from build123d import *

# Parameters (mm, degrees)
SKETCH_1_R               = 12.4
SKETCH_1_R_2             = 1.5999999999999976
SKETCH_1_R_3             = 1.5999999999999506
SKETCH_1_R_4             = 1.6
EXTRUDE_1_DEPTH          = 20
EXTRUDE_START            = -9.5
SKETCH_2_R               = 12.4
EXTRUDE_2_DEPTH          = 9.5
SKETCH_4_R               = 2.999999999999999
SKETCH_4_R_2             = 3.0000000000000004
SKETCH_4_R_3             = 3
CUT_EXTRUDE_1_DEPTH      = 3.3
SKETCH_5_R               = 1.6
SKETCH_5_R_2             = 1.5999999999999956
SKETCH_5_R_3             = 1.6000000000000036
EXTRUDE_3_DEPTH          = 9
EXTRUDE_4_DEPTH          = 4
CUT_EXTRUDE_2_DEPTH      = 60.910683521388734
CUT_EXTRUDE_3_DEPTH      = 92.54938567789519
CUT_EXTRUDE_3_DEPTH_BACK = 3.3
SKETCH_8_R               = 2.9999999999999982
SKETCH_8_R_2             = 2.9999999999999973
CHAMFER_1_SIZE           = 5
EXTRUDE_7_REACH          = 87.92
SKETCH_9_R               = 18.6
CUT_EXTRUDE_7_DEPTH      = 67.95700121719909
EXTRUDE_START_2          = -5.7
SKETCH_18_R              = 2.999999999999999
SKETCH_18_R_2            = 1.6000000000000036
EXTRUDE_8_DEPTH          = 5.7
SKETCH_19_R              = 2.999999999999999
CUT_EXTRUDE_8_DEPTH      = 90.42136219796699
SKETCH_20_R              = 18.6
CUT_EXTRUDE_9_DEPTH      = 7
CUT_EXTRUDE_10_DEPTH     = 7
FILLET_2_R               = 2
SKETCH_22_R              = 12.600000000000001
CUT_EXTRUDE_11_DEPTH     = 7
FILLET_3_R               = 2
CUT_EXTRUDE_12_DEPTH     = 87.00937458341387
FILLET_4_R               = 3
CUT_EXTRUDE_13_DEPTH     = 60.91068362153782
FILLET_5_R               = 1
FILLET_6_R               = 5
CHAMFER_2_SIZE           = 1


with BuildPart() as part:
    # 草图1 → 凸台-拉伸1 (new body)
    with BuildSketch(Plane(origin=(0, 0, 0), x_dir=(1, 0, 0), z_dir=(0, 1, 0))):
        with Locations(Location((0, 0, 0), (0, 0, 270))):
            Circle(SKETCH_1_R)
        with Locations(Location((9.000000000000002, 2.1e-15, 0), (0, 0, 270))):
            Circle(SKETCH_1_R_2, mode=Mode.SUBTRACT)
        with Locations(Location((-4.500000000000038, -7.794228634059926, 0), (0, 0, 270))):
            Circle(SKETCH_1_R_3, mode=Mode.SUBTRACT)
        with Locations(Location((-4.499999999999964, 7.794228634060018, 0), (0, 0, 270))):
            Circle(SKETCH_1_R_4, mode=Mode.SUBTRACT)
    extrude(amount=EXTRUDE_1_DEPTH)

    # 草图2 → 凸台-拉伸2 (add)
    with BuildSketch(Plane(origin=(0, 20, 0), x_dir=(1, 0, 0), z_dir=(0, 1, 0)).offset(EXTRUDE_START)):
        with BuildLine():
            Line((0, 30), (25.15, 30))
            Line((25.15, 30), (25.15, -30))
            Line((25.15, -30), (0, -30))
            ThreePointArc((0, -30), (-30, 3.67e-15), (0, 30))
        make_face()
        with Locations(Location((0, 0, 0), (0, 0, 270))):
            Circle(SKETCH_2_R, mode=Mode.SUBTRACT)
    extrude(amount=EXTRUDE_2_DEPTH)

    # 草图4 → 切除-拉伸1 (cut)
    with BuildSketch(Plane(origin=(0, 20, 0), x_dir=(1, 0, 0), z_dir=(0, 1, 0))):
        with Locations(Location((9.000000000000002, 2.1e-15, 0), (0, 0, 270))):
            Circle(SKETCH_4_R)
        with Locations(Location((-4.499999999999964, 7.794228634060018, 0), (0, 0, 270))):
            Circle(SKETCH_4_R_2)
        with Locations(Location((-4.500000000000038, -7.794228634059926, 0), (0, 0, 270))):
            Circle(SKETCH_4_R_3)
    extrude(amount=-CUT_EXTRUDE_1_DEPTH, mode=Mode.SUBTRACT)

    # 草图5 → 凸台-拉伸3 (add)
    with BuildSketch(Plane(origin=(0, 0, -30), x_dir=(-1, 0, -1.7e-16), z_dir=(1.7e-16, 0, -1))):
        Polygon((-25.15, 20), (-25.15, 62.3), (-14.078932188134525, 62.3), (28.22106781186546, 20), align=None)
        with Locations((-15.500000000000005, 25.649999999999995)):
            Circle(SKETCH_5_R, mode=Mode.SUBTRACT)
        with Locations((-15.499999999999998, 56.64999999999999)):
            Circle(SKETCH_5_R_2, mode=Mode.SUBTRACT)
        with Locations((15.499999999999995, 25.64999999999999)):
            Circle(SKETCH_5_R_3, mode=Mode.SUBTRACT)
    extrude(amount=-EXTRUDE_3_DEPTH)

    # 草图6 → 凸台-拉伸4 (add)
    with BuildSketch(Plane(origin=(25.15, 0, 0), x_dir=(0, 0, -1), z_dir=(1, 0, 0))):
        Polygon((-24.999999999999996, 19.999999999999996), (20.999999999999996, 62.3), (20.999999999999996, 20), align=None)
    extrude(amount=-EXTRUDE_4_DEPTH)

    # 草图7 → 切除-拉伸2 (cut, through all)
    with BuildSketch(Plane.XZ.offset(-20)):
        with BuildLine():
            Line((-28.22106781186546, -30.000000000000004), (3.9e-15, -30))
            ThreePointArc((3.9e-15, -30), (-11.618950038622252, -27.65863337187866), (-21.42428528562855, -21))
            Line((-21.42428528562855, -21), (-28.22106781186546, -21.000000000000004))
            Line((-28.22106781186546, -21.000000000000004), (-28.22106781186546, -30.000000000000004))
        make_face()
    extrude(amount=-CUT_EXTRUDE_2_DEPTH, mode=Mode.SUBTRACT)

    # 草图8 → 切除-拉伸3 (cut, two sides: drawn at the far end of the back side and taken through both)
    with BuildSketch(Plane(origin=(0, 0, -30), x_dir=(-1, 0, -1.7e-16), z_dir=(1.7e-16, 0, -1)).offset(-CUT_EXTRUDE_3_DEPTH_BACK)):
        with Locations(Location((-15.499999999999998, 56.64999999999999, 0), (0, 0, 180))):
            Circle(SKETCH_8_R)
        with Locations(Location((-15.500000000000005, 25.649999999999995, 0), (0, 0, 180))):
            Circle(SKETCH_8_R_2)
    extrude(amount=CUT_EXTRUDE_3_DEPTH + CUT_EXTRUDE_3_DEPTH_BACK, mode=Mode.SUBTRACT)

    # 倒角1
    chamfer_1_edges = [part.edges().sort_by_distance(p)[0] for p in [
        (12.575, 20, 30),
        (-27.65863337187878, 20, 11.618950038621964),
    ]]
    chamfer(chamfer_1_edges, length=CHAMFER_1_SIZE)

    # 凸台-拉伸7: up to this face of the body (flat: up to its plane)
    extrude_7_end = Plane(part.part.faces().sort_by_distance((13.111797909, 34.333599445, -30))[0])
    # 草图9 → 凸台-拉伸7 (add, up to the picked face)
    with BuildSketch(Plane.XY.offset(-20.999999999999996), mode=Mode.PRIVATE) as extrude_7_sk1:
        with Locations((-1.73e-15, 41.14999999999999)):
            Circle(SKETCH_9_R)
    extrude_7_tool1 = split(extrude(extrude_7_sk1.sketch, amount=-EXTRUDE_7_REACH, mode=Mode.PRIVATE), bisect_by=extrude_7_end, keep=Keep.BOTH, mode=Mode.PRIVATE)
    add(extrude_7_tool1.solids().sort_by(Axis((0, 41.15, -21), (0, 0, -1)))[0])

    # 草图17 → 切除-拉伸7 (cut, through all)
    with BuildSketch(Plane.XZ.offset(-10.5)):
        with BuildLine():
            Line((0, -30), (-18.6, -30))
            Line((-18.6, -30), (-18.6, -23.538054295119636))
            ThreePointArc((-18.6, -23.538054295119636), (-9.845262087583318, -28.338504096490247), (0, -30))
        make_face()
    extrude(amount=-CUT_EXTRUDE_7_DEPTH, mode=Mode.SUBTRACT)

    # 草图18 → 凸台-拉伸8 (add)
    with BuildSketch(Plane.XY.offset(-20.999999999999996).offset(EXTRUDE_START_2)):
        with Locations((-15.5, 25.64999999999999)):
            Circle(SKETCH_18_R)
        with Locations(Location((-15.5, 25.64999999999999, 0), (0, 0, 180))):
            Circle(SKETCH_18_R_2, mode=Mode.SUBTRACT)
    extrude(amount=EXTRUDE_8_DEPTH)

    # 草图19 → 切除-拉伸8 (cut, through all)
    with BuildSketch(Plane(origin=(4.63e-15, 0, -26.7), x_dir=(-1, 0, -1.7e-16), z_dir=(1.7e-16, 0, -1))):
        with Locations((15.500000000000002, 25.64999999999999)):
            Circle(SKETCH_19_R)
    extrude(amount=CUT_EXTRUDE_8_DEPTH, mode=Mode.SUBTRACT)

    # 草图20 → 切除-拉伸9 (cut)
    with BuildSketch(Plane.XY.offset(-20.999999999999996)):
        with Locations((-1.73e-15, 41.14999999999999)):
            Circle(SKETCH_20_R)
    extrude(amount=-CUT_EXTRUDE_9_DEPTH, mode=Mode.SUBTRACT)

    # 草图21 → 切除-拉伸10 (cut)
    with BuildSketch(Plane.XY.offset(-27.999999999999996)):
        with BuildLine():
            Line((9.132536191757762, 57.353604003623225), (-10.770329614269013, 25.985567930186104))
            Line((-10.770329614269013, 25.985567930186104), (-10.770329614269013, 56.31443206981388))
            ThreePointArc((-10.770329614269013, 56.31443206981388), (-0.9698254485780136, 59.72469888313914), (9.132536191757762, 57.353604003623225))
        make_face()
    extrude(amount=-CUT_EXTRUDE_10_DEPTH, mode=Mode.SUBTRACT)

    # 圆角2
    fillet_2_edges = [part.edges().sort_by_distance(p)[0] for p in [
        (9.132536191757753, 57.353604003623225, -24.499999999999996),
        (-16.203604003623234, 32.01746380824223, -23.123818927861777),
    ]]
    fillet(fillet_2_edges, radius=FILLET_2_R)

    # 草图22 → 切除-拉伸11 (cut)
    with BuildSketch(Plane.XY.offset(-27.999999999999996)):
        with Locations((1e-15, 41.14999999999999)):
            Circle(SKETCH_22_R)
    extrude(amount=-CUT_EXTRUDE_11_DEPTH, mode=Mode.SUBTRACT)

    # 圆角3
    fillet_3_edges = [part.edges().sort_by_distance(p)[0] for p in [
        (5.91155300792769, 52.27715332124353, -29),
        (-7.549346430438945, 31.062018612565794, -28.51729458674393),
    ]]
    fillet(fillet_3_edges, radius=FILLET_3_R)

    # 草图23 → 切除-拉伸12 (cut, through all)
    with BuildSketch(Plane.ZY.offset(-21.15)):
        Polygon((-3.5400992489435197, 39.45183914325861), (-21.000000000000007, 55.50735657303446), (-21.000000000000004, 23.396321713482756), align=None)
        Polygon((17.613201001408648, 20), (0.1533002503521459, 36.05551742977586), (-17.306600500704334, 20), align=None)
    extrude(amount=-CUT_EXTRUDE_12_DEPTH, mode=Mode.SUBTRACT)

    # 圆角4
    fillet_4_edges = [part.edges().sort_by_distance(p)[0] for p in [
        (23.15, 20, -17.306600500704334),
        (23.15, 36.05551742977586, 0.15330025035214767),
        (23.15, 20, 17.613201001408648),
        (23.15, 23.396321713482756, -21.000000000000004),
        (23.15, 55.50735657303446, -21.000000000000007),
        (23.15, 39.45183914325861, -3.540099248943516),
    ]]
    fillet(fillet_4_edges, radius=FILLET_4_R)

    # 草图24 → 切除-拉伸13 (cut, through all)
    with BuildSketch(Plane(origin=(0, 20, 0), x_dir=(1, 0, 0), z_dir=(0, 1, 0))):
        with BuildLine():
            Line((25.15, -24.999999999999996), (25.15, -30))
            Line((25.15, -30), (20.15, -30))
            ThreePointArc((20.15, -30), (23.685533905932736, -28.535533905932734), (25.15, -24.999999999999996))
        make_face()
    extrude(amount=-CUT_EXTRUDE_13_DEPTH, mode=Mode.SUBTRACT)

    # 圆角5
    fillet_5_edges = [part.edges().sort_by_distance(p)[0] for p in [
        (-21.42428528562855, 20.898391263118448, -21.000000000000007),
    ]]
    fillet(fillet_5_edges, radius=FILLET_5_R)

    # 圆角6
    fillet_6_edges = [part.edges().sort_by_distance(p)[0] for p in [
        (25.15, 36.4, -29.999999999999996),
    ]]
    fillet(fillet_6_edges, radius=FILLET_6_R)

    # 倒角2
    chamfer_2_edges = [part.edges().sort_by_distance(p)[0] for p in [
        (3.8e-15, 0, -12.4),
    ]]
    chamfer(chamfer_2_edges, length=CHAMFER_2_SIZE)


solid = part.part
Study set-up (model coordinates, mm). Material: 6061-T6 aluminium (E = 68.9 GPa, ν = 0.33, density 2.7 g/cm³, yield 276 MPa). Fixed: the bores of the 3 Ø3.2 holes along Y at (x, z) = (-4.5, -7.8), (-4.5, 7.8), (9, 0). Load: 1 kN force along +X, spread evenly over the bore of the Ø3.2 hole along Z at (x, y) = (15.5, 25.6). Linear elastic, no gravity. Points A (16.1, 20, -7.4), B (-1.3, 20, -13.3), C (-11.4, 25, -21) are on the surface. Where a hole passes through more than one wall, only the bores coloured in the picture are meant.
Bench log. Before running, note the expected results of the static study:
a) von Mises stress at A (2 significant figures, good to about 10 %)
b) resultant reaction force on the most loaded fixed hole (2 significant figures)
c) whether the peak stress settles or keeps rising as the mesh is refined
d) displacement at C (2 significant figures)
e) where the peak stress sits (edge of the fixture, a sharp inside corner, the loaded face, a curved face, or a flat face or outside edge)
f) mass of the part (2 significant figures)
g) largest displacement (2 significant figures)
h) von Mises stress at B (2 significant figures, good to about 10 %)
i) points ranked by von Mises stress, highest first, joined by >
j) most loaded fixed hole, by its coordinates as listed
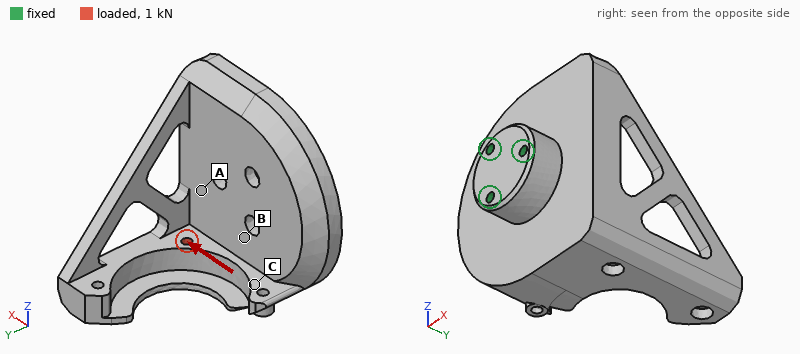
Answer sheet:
9.6 MPa
1.2 kN
keeps rising
8.2 µm
edge of the fixture
100 g
45 µm
13 MPa
B > A > C
(-4.5, -7.8)
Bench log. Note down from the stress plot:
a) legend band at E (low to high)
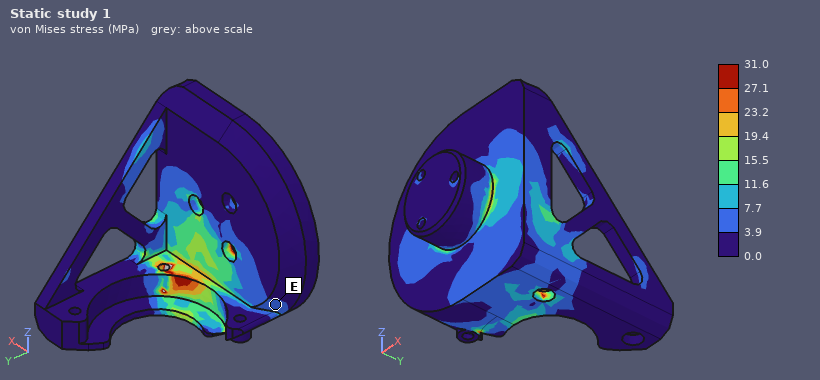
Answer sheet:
3.9 to 7.7 MPa
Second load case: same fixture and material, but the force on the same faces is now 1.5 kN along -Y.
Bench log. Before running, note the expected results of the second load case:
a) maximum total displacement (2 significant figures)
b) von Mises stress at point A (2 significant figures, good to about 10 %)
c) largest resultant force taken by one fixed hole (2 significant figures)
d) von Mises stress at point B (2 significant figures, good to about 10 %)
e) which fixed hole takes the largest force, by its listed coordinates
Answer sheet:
89 µm
27 MPa
1.3 kN
21 MPa
(9, 0)
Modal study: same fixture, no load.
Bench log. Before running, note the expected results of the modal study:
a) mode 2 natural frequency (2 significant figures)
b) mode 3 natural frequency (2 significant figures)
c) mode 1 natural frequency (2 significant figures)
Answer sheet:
4600 Hz
6800 Hz
3400 Hz
